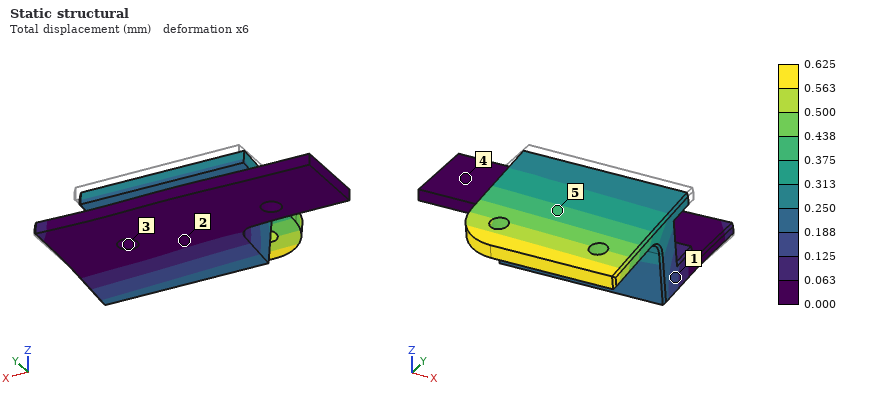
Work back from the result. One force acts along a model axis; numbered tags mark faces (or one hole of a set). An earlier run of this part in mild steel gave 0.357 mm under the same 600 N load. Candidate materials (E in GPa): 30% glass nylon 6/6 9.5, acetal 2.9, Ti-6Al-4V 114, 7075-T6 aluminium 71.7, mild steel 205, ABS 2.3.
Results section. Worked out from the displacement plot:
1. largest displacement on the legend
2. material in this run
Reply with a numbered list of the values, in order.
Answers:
1. 0.625 mm
2. Ti-6Al-4V
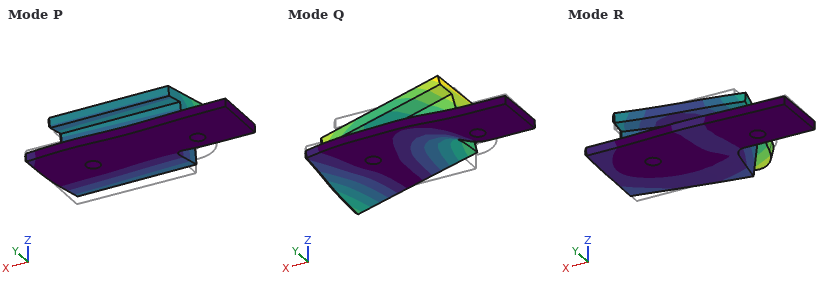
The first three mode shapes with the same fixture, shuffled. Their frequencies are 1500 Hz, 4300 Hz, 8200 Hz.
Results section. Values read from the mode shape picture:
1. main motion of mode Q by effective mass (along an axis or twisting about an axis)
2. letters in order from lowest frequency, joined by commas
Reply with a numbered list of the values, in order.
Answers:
1. along X
2. P, Q, R
